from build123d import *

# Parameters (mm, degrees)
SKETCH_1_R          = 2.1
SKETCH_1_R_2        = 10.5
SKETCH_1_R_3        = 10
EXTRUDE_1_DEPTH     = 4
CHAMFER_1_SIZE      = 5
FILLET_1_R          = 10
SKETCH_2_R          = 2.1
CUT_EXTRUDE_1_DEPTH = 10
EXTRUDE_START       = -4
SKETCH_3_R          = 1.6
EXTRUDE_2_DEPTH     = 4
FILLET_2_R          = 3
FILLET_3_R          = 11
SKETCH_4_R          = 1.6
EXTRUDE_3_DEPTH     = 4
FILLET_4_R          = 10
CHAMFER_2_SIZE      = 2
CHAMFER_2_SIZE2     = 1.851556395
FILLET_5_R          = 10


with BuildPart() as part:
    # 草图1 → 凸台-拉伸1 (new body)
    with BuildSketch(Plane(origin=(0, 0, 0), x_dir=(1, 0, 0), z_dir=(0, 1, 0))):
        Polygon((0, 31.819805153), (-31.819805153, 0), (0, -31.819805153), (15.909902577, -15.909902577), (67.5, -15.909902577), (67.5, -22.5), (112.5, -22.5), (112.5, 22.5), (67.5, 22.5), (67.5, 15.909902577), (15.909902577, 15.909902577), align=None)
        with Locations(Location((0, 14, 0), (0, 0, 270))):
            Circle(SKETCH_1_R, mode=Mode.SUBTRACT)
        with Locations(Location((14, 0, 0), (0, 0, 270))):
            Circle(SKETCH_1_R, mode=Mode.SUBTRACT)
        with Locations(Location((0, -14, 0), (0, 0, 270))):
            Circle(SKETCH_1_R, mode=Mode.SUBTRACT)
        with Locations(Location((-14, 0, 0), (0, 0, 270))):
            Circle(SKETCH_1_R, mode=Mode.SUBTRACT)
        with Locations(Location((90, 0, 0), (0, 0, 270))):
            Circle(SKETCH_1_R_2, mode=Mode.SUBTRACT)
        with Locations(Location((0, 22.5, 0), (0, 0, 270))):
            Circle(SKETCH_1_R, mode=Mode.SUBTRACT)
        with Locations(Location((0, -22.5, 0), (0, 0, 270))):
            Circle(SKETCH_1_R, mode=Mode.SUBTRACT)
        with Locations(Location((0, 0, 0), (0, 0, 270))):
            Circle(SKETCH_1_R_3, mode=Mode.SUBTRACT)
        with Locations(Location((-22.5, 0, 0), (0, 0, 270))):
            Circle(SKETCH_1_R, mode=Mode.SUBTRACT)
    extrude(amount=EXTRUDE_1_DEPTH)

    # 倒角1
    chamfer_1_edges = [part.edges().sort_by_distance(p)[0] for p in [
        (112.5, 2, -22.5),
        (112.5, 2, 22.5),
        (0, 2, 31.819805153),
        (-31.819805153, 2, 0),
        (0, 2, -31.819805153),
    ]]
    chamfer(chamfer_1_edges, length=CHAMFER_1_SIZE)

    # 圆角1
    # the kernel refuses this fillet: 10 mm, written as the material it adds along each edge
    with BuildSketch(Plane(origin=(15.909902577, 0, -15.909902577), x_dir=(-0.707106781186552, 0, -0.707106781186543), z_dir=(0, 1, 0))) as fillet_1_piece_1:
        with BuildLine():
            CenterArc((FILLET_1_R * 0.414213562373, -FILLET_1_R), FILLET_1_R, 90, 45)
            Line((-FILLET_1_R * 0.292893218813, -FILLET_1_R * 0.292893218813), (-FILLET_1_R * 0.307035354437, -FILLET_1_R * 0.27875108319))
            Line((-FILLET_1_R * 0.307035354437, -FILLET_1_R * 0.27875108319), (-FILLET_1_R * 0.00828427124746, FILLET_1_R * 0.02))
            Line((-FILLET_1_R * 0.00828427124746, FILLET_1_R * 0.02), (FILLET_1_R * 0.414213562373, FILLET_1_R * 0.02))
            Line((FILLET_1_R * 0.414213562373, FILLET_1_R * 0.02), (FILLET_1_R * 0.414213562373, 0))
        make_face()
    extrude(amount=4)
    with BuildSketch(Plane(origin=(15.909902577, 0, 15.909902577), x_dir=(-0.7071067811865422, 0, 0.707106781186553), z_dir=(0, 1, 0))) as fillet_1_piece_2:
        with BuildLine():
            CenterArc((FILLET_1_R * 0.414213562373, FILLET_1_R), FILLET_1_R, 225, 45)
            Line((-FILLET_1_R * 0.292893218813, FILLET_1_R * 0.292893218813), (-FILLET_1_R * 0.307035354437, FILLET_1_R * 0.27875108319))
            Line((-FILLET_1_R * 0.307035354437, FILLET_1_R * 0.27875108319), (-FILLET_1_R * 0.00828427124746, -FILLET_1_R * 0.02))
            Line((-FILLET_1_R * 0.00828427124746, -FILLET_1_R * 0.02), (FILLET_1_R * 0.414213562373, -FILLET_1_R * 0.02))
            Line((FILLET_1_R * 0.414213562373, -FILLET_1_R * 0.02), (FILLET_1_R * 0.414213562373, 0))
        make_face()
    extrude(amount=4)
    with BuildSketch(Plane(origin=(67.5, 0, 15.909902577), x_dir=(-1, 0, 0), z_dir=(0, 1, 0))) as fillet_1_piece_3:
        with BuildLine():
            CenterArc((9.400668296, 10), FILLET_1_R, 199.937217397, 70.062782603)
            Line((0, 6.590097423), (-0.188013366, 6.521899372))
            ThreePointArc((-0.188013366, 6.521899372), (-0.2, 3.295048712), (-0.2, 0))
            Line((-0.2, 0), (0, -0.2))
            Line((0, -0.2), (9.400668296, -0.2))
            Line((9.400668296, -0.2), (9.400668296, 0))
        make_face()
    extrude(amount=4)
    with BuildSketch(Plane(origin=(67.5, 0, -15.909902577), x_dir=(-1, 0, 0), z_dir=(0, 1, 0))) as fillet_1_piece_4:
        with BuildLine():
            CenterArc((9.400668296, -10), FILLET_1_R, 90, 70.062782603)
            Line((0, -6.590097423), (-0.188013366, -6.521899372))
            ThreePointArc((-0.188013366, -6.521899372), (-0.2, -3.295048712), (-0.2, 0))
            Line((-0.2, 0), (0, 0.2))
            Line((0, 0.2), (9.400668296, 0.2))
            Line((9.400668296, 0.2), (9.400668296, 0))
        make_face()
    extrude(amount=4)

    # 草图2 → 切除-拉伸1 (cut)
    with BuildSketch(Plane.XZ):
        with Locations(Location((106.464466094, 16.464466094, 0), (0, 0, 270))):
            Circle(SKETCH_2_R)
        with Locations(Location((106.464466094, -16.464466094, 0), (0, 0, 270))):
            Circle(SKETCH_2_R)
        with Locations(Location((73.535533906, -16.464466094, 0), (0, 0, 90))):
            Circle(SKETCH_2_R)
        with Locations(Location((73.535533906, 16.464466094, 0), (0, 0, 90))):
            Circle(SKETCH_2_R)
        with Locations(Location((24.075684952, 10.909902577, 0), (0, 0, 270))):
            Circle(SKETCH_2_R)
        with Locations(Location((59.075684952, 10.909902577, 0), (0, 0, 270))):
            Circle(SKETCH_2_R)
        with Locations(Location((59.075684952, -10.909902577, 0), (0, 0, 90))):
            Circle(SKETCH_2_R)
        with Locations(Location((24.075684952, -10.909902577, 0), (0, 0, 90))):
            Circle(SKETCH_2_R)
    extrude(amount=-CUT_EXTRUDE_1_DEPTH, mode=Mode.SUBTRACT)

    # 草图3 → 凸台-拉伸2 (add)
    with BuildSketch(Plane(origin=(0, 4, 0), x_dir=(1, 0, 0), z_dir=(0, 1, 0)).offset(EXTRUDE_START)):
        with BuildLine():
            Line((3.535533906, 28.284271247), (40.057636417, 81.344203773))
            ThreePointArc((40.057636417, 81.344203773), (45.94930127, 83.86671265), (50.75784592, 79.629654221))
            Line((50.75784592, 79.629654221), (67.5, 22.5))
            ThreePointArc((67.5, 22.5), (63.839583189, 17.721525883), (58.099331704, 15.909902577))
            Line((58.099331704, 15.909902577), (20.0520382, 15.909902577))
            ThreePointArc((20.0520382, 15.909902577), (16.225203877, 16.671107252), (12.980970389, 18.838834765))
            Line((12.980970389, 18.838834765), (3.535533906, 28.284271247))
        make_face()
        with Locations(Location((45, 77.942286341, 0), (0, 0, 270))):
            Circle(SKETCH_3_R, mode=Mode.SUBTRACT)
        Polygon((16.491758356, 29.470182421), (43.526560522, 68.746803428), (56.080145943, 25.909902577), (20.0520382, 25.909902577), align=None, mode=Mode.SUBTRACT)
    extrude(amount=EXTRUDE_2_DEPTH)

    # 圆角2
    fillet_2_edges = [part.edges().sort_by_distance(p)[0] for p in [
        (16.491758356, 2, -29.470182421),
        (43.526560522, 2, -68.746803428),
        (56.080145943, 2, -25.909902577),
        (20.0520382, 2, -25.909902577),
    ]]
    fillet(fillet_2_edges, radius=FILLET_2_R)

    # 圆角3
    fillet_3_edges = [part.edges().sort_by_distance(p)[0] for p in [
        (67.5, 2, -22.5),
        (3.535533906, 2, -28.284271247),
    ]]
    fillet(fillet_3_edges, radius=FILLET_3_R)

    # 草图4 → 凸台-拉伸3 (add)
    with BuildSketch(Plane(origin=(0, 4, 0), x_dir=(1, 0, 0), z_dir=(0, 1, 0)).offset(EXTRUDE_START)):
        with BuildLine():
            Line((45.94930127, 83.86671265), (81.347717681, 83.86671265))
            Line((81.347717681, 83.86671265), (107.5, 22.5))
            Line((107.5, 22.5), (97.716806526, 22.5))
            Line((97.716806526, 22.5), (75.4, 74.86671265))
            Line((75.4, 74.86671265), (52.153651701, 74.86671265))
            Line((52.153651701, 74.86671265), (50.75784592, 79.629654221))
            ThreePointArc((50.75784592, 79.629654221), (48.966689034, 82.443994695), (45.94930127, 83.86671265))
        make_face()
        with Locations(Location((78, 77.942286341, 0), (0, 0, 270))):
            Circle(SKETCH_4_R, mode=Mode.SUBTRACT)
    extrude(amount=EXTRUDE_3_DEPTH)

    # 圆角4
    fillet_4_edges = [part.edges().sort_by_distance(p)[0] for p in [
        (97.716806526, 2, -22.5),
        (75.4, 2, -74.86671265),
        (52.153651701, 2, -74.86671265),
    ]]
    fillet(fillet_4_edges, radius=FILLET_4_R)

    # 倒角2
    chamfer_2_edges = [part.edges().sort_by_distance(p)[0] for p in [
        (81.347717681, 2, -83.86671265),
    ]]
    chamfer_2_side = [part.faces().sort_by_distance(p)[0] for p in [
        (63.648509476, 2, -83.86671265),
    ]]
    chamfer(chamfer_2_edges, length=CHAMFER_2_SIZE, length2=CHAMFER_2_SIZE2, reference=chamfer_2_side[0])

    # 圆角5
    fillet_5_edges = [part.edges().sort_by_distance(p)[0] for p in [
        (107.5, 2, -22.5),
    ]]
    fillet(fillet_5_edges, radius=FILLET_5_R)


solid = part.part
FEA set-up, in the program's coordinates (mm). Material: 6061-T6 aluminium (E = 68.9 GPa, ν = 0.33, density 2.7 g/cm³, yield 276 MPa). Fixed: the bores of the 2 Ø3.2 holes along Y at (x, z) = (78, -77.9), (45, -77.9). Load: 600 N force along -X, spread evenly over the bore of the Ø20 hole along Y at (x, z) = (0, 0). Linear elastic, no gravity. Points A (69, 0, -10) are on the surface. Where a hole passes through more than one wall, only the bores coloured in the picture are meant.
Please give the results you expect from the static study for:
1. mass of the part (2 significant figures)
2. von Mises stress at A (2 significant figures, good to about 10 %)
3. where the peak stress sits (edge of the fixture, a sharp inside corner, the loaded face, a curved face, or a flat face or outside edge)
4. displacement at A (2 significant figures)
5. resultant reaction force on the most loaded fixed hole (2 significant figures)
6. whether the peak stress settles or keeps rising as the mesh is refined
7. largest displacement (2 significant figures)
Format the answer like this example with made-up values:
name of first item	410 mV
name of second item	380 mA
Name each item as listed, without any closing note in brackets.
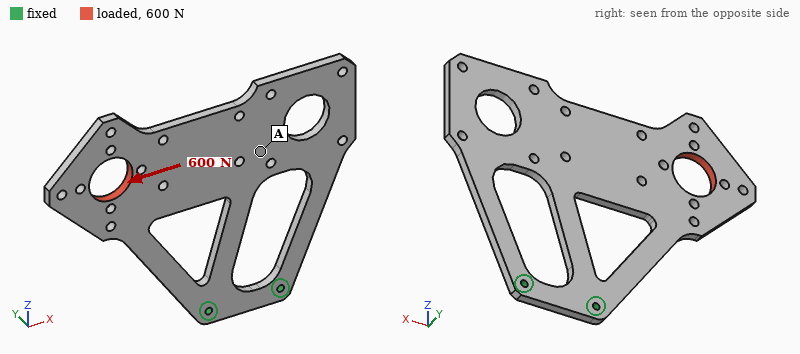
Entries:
mass of the part	78 g
von Mises stress at A	15 MPa
where the peak stress sits	edge of the fixture
displacement at A	0.23 mm
resultant reaction force on the most loaded fixed hole	1.4 kN
whether the peak stress settles or keeps rising as the mesh is refined	keeps rising
largest displacement	0.37 mm
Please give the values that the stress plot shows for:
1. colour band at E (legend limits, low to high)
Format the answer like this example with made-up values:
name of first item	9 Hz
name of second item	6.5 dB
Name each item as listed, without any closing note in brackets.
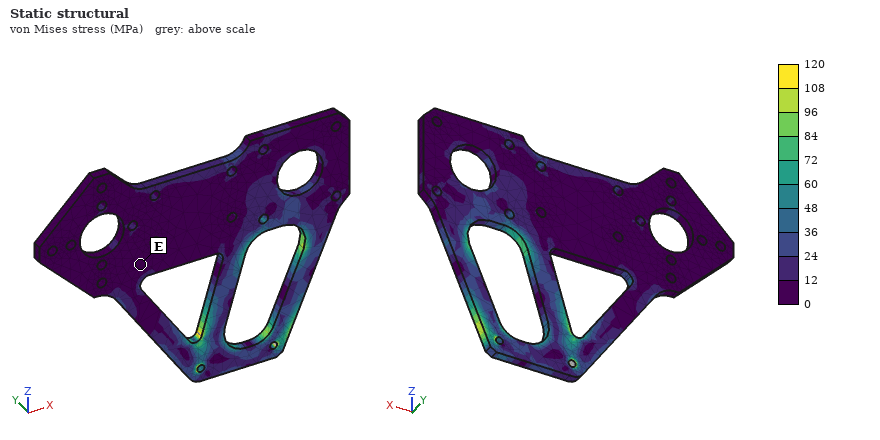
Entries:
colour band at E	0 to 12 MPa
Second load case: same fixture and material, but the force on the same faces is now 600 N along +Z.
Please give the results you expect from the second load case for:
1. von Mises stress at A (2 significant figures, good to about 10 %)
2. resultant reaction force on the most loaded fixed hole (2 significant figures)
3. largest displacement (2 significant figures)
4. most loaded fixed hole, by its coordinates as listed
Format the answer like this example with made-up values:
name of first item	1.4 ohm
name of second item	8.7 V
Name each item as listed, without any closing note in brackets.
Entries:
von Mises stress at A	9.4 MPa
resultant reaction force on the most loaded fixed hole	1.3 kN
largest displacement	0.23 mm
most loaded fixed hole, by its coordinates as listed	(45, -77.9)
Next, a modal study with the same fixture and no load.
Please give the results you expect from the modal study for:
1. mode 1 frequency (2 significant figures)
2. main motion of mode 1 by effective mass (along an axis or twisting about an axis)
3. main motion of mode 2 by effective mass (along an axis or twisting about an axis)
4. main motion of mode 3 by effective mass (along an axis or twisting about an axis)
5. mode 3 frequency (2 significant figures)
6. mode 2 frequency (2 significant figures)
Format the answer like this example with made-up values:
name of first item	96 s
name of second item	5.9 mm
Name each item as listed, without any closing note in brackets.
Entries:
mode 1 frequency	170 Hz
main motion of mode 1 by effective mass	along Y
main motion of mode 2 by effective mass	twisting about Z
main motion of mode 3 by effective mass	along X
mode 3 frequency	950 Hz
mode 2 frequency	330 Hz
